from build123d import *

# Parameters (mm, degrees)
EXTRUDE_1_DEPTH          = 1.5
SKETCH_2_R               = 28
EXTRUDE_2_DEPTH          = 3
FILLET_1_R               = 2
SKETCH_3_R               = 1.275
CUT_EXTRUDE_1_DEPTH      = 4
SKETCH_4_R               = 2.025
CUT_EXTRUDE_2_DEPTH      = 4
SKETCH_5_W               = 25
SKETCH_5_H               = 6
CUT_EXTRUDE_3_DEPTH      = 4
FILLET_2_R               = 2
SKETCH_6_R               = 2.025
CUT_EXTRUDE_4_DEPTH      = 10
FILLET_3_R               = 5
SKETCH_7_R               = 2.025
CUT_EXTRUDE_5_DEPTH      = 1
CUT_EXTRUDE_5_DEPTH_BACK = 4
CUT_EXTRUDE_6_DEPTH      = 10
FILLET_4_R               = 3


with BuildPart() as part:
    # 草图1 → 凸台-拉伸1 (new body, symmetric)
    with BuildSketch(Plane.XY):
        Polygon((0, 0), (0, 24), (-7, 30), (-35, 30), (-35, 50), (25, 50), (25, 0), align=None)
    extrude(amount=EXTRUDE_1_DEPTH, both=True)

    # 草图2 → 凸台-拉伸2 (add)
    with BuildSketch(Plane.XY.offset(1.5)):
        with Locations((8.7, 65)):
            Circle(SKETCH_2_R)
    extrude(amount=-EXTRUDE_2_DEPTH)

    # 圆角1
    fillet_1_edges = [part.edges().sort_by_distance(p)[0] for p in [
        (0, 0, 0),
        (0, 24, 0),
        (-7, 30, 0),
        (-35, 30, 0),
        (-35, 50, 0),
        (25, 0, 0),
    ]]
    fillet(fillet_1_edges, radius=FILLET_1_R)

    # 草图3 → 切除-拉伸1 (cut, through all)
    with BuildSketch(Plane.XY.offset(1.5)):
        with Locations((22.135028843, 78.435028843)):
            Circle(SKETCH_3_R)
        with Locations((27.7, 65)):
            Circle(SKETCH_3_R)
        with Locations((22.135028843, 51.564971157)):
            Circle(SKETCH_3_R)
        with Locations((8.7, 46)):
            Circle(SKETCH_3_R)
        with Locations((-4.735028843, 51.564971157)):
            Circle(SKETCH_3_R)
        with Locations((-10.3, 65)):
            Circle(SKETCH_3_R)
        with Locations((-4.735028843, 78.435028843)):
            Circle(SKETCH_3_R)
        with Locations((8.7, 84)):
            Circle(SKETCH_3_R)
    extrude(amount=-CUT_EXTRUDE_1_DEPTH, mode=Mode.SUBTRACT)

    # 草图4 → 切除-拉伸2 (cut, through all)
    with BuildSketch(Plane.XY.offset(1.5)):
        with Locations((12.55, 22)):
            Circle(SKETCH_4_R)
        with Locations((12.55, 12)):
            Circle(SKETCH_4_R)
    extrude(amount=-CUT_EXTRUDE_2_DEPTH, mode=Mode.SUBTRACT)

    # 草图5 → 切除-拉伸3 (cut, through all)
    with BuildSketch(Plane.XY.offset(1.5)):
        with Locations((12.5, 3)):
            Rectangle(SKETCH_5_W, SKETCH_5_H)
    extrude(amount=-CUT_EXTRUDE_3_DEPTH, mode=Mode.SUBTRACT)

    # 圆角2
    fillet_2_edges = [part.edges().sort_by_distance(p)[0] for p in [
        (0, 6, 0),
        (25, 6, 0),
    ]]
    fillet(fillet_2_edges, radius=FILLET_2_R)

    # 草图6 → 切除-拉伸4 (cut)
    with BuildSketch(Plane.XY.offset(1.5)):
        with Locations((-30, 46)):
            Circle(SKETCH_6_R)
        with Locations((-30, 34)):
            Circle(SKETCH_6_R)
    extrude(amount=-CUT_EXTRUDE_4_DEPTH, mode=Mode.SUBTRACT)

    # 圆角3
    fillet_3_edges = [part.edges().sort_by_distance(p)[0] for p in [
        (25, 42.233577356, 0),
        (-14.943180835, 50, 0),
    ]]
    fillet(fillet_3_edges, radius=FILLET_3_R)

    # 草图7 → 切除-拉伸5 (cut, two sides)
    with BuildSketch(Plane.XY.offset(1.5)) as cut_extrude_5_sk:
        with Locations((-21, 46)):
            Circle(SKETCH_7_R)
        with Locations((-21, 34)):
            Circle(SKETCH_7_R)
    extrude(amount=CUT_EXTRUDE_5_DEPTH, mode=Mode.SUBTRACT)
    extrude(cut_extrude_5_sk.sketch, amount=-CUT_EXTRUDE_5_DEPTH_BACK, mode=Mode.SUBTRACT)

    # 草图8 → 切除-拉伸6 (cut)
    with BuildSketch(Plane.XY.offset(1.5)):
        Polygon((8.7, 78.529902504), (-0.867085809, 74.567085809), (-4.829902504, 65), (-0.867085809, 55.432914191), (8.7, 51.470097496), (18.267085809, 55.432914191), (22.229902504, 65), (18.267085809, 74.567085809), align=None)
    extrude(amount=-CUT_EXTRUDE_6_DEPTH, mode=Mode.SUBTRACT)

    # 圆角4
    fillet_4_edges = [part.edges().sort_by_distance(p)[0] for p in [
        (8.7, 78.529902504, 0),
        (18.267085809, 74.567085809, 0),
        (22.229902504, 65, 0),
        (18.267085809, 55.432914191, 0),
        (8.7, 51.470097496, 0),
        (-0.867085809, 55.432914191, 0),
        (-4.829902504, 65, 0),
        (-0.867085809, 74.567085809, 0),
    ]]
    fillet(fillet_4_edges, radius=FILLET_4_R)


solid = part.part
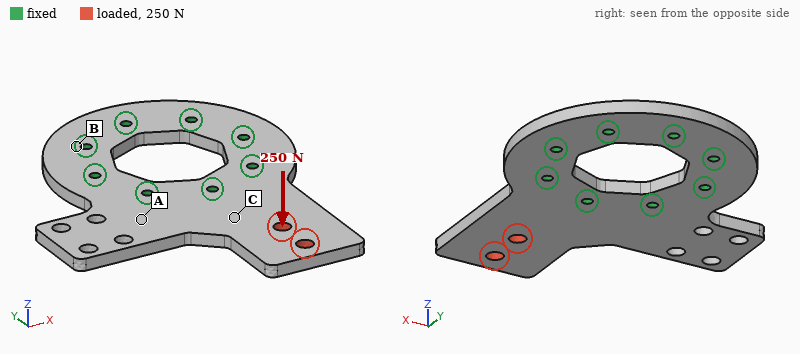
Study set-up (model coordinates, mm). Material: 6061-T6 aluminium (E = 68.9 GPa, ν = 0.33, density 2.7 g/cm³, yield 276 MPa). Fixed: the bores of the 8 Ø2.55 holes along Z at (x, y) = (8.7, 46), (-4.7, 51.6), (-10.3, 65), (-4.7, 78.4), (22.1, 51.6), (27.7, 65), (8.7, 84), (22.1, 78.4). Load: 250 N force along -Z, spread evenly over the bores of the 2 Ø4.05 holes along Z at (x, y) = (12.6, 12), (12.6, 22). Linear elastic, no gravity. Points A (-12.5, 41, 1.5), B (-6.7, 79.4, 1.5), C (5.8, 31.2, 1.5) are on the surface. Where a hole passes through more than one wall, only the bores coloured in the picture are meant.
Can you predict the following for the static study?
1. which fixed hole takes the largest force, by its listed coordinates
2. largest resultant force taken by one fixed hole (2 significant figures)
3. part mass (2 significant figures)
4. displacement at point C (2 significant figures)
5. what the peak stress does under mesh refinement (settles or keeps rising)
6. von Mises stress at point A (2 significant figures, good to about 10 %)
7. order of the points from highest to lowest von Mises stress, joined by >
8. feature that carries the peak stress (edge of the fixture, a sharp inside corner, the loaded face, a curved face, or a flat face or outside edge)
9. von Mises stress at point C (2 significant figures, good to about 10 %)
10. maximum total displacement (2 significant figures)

(8.7, 46)
420 N
26 g
0.14 mm
keeps rising
38 MPa
C > A > B
edge of the fixture
77 MPa
0.72 mm
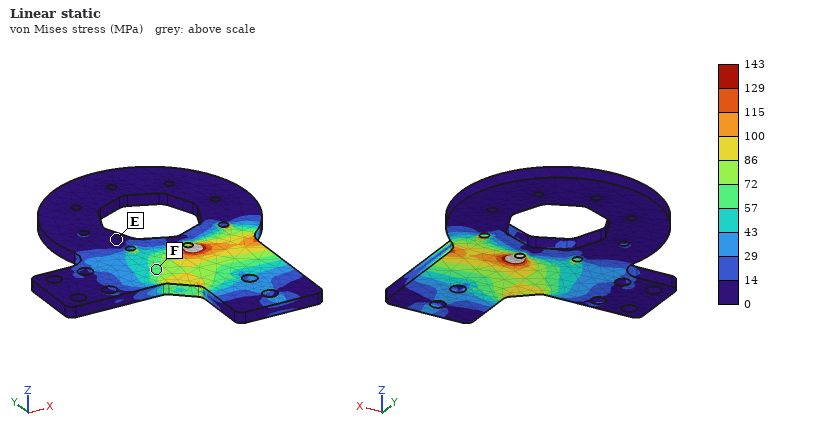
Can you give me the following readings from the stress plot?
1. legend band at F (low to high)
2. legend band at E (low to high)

57 to 72 MPa
0 to 14 MPa
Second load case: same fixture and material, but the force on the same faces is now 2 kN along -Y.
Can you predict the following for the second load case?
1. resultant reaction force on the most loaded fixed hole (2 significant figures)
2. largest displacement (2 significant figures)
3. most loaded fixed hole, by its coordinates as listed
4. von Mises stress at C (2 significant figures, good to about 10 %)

870 N
18 µm
(8.7, 46)
24 MPa
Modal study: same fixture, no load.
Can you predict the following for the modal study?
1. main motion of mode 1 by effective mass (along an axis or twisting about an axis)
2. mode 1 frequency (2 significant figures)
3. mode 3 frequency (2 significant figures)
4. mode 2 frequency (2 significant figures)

along Z
1700 Hz
5200 Hz
2600 Hz
